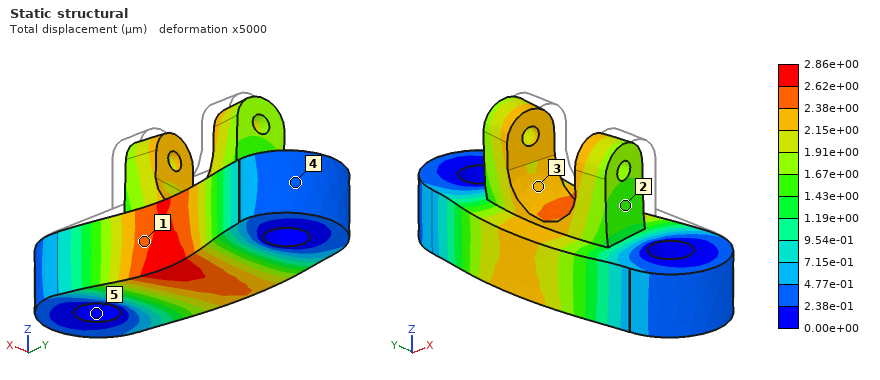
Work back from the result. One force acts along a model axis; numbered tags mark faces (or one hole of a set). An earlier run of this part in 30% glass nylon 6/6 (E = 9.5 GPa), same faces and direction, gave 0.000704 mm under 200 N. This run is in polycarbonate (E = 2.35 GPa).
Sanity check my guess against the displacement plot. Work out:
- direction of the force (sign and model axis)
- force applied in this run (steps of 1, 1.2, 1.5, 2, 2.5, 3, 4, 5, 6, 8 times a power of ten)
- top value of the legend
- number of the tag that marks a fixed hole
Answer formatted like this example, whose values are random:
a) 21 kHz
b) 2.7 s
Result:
a) -X
b) 200 N
c) 2.86e+00 µm
d) 5
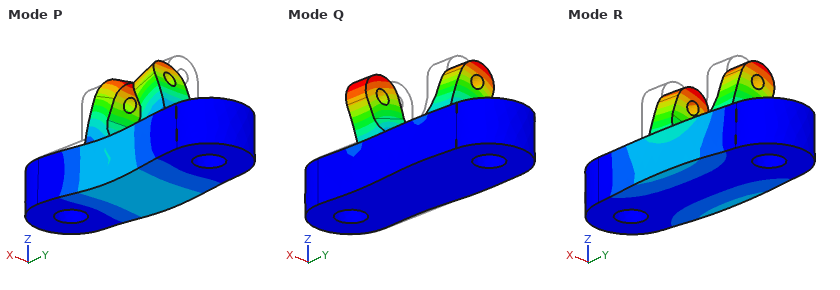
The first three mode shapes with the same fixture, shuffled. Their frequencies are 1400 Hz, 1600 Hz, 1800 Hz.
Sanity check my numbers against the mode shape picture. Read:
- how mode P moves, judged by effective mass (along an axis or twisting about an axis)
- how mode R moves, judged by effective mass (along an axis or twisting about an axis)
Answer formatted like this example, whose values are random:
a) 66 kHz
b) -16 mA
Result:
a) along Z
b) along X
